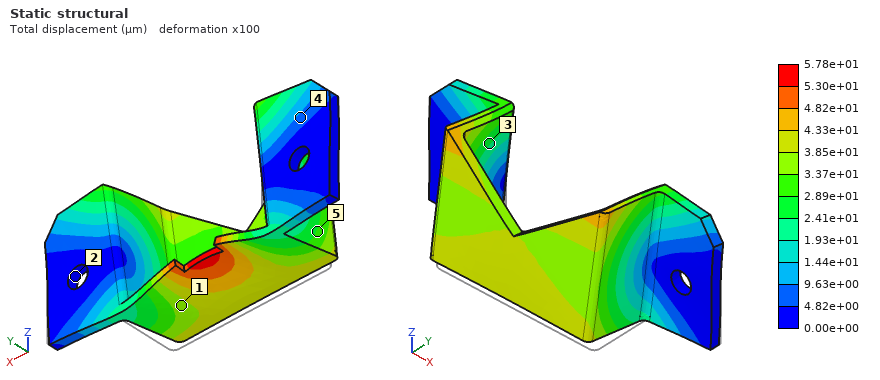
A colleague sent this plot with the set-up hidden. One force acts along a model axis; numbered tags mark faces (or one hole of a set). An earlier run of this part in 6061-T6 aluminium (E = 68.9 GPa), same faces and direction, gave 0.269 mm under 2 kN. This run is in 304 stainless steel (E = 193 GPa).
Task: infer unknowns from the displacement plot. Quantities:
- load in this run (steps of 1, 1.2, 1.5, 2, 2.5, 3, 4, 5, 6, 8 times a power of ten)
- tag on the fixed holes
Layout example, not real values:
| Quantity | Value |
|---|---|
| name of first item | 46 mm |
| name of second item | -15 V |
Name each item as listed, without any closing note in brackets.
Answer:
| Quantity | Value |
|---|---|
| load in this run | 1.2 kN |
| tag on the fixed holes | 2 |
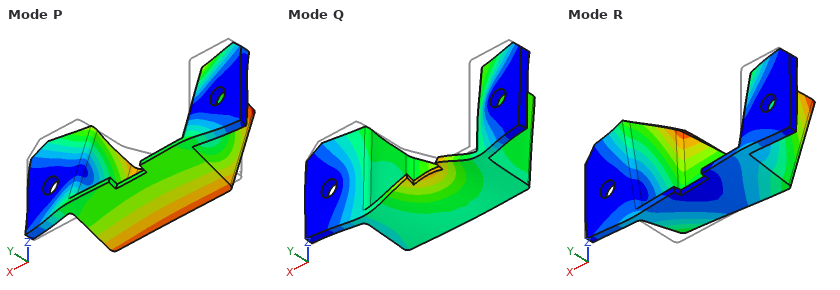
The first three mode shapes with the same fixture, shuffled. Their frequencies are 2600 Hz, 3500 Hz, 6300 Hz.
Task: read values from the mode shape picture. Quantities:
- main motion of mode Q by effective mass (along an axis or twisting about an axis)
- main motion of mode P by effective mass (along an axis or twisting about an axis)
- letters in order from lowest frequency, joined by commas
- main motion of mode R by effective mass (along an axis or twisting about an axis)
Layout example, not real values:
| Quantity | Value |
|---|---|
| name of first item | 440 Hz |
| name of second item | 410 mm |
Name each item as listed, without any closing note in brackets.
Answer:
| Quantity | Value |
|---|---|
| main motion of mode Q by effective mass | along Y |
| main motion of mode P by effective mass | along Z |
| letters in order from lowest frequency, joined by commas | P, R, Q |
| main motion of mode R by effective mass | along X |
